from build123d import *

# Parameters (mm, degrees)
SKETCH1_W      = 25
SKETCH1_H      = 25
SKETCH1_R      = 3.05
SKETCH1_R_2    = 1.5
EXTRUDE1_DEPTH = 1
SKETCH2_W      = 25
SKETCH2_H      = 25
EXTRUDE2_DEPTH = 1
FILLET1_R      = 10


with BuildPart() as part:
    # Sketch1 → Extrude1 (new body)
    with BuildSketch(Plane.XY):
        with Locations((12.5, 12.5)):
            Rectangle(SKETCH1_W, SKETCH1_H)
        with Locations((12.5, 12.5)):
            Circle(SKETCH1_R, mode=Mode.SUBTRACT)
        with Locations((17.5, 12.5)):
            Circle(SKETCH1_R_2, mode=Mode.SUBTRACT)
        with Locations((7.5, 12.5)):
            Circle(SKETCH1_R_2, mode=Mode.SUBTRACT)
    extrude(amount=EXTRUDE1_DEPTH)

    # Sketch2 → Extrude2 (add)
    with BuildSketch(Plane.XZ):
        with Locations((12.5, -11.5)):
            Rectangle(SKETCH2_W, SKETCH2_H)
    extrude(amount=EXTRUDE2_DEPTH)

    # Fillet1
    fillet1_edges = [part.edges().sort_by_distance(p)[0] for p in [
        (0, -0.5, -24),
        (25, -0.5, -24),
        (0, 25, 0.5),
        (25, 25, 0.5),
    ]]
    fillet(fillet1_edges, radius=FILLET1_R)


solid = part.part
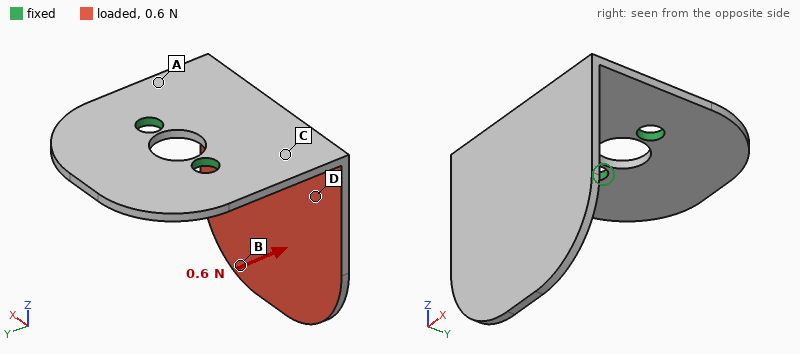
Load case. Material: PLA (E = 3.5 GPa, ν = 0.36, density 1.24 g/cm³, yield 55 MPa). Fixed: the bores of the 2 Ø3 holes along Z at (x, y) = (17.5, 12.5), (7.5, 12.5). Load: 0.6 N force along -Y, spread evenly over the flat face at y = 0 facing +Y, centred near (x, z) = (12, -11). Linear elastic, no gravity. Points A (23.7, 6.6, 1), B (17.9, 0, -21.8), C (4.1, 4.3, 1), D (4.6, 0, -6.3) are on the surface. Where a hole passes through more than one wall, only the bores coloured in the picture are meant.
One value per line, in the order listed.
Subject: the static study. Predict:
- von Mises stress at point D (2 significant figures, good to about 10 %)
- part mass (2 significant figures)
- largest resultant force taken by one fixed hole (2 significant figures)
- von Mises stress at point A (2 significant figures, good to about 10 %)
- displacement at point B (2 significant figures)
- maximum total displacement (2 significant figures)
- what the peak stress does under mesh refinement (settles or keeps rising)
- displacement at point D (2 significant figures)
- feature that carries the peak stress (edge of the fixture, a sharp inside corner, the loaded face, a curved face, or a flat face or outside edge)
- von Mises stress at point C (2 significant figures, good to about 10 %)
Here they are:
0.76 MPa
1.4 g
0.31 N
1.7 MPa
0.37 mm
0.41 mm
keeps rising
0.12 mm
edge of the fixture
1.5 MPa
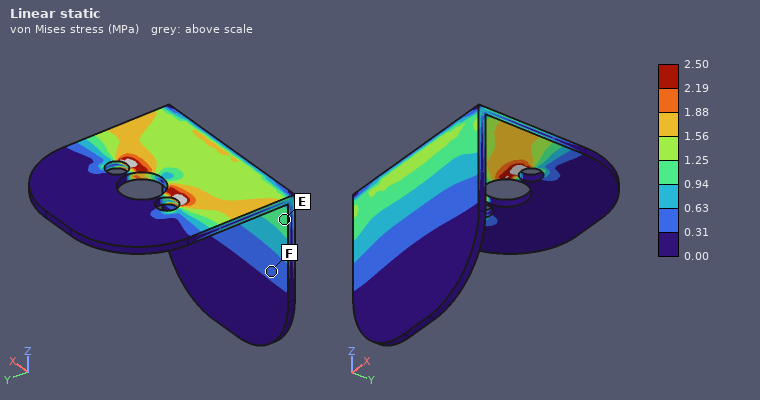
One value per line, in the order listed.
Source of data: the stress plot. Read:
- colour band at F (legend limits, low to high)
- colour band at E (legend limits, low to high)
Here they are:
0.31 to 0.63 MPa
0.94 to 1.25 MPa
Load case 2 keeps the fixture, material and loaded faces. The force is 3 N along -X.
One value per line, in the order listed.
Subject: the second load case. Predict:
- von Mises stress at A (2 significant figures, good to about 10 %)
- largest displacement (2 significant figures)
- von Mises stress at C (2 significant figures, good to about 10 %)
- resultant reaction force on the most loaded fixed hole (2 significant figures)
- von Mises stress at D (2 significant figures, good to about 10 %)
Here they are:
3.4 MPa
0.48 mm
3.0 MPa
3.8 N
1.8 MPa
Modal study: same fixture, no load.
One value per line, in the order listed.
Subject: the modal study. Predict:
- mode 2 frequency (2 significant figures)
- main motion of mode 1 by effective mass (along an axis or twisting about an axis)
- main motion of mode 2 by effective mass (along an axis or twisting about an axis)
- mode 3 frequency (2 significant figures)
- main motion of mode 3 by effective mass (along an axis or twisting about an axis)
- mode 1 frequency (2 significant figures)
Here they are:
530 Hz
along Y
along X
900 Hz
along Z
280 Hz
